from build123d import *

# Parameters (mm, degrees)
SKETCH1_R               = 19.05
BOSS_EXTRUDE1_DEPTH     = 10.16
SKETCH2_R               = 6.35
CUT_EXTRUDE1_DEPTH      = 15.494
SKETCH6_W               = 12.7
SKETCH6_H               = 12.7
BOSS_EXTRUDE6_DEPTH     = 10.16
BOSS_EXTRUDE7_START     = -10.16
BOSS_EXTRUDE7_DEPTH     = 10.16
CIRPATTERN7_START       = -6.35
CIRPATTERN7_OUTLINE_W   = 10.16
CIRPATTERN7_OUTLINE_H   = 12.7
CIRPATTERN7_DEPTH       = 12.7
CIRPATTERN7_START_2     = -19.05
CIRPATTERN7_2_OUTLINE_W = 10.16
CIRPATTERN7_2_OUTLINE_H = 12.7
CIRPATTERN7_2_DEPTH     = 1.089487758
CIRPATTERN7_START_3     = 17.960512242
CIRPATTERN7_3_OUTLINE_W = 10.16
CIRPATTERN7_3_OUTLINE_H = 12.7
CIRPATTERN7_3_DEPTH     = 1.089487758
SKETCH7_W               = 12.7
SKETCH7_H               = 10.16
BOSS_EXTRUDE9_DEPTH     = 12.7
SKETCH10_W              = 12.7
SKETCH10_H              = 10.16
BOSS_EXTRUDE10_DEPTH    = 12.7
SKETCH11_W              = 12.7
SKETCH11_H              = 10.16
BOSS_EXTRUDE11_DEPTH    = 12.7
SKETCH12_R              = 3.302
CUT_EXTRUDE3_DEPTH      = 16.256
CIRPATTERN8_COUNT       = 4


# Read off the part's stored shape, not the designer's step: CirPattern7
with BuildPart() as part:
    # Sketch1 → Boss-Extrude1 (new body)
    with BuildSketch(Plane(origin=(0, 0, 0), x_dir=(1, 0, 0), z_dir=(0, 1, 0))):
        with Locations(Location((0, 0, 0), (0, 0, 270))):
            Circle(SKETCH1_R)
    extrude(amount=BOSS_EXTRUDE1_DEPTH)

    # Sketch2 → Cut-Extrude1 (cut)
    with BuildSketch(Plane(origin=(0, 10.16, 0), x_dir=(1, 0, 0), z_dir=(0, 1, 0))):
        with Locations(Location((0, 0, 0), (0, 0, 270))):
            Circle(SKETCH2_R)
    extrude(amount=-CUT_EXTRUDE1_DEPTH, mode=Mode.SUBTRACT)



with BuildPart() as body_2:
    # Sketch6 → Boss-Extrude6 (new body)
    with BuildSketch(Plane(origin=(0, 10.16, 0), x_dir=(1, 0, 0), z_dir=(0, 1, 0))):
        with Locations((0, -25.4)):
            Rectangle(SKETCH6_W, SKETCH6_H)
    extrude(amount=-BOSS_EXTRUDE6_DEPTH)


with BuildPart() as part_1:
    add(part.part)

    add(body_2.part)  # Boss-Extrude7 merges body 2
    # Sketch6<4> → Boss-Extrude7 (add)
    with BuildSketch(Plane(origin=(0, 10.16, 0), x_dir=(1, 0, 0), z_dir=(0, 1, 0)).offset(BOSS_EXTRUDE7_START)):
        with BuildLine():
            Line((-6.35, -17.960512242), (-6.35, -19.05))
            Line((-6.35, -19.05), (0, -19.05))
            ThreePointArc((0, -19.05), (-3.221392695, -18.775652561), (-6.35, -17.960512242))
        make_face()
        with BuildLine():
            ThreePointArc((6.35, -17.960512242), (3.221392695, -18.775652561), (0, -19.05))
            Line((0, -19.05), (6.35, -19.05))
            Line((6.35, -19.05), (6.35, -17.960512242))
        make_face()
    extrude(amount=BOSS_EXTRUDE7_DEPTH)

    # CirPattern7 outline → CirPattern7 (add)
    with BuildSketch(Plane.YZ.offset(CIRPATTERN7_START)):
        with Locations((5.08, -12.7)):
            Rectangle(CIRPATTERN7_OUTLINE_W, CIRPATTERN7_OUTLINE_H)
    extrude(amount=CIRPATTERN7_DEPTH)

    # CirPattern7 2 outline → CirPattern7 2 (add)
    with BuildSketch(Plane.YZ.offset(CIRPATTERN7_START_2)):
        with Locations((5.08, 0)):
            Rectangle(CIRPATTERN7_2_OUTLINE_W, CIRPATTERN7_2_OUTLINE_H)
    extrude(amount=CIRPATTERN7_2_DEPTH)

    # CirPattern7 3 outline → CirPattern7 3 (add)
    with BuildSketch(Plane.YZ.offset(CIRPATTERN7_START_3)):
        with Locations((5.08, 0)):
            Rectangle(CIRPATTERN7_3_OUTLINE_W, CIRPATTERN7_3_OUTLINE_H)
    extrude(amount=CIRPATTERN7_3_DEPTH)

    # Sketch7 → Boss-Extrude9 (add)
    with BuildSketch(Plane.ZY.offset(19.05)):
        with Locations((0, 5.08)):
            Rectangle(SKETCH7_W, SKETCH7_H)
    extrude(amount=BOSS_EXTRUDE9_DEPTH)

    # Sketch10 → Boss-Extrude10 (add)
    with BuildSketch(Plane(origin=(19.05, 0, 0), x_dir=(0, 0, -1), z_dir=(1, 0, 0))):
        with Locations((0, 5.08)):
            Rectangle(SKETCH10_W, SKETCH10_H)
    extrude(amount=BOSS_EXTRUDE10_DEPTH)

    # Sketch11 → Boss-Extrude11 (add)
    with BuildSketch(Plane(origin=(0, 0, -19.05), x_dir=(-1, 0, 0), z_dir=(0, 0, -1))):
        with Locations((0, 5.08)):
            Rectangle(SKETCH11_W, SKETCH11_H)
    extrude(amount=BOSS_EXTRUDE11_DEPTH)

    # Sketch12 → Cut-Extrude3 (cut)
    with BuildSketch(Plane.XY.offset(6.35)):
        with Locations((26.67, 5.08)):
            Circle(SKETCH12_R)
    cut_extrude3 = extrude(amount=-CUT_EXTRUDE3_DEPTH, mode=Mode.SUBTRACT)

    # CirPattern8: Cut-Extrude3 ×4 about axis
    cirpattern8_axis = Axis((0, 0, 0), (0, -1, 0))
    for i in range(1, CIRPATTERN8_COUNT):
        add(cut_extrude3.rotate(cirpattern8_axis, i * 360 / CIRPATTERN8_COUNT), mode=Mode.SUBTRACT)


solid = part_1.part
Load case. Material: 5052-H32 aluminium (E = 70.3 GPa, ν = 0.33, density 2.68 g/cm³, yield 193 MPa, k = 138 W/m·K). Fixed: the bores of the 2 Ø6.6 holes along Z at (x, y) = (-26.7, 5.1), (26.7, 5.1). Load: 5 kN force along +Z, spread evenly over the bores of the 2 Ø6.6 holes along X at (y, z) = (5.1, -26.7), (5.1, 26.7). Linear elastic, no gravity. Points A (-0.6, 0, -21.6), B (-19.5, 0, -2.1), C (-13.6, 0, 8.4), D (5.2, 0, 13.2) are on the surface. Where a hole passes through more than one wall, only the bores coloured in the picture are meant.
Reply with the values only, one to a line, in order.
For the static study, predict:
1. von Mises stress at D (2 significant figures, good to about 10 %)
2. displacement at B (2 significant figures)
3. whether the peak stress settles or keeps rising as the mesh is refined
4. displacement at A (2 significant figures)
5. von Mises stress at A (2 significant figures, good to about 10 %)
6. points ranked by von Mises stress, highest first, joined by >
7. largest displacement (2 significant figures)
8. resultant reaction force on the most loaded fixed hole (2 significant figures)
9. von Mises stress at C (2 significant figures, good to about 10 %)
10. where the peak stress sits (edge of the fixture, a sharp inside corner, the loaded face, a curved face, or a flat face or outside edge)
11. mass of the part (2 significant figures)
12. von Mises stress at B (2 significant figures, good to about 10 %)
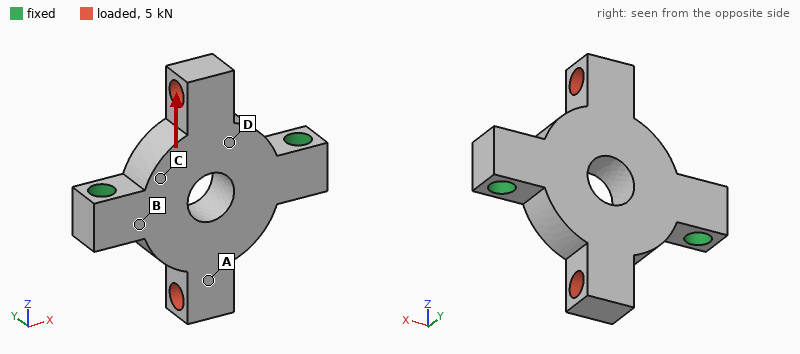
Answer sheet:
15 MPa
4.6 µm
keeps rising
15 µm
33 MPa
B > A > C > D
23 µm
2.5 kN
21 MPa
edge of the fixture
41 g
41 MPa
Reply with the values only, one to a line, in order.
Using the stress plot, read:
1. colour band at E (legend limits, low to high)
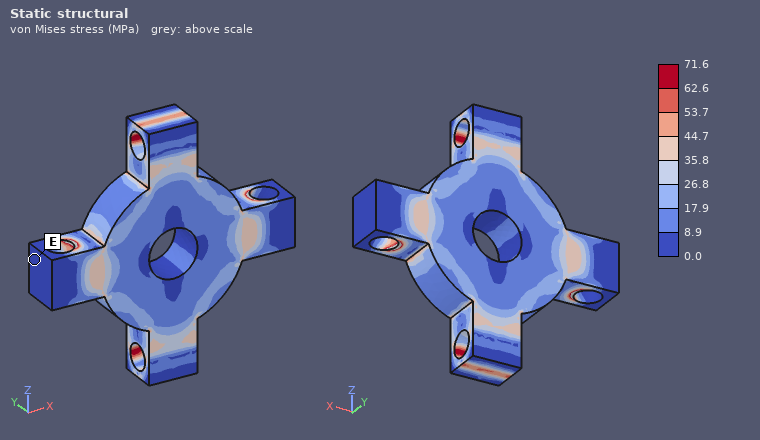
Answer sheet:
0.0 to 8.9 MPa
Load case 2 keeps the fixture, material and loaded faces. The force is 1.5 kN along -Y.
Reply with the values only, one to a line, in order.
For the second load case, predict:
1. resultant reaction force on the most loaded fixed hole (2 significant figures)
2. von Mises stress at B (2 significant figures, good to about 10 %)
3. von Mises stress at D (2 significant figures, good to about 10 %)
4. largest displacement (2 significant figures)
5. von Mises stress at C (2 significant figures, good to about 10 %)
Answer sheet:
750 N
24 MPa
42 MPa
78 µm
29 MPa
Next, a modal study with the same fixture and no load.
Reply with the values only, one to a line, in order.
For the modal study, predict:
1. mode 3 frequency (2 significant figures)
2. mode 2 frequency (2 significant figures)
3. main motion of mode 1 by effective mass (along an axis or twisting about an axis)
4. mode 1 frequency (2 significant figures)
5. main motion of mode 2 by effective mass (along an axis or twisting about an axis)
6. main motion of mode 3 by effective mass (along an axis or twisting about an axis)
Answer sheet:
18 kHz
8300 Hz
twisting about X
6000 Hz
along Y
along Z
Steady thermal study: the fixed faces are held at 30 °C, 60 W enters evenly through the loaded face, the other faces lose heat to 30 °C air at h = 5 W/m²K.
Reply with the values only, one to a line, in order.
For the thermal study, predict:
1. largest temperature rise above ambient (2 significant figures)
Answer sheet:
58 K
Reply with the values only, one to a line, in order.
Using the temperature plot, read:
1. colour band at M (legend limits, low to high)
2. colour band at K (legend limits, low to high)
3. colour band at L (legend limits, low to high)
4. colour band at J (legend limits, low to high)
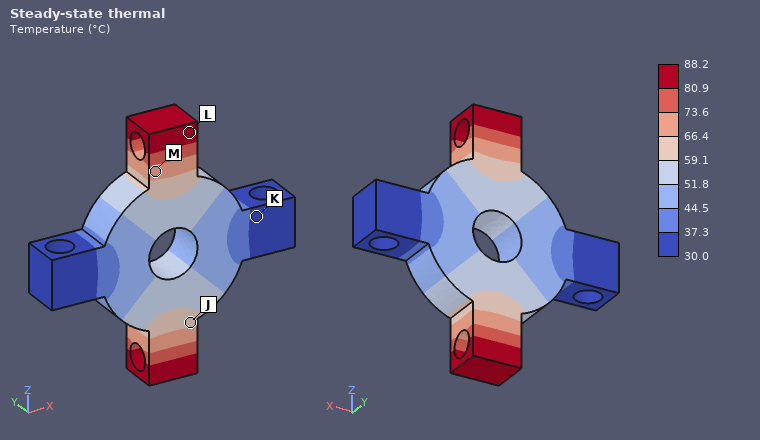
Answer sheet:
66.4 to 73.6 °C
30.0 to 37.3 °C
80.9 to 88.2 °C
59.1 to 66.4 °C
